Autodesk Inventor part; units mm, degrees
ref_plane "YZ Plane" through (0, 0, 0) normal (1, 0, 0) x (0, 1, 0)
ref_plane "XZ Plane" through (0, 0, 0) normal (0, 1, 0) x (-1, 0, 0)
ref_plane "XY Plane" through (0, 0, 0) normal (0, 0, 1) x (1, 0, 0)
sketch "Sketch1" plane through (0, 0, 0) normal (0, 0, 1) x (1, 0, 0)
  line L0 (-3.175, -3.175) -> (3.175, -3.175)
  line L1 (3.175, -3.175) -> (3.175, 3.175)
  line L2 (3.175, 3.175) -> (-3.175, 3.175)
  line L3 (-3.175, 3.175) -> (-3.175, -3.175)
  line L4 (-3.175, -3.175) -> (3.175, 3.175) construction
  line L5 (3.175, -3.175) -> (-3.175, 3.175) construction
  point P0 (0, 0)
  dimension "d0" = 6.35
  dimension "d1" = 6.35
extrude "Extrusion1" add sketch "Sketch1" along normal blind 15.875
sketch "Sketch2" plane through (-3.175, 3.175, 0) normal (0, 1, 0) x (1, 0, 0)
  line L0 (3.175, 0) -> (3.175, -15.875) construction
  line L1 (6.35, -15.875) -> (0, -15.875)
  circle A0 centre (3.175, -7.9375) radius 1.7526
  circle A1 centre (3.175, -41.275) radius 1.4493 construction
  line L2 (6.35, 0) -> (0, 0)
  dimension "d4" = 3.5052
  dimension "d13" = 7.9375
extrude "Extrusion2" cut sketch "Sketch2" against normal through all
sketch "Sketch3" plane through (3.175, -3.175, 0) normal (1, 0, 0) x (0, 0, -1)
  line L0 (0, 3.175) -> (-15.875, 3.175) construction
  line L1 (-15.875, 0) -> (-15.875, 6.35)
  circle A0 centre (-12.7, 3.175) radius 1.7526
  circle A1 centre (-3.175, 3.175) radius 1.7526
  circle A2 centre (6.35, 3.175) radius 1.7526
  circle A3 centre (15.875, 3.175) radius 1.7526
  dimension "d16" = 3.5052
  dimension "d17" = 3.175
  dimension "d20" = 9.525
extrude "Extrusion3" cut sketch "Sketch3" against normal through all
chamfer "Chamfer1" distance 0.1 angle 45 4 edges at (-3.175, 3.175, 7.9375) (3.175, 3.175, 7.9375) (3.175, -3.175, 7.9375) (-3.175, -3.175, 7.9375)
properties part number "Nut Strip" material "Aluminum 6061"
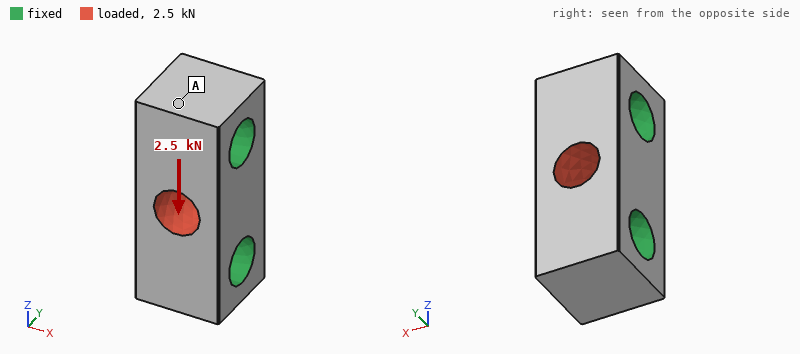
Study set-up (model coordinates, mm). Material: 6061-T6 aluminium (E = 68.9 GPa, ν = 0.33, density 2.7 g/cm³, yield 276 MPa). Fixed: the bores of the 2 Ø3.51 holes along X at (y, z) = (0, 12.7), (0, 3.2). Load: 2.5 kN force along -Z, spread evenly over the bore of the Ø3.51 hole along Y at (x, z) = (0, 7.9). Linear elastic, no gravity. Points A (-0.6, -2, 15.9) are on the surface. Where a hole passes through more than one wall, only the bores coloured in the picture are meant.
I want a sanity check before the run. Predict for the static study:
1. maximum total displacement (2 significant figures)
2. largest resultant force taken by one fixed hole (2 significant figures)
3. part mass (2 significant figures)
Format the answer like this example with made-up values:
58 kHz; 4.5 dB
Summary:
1.9 µm; 1.3 kN; 1.2 g
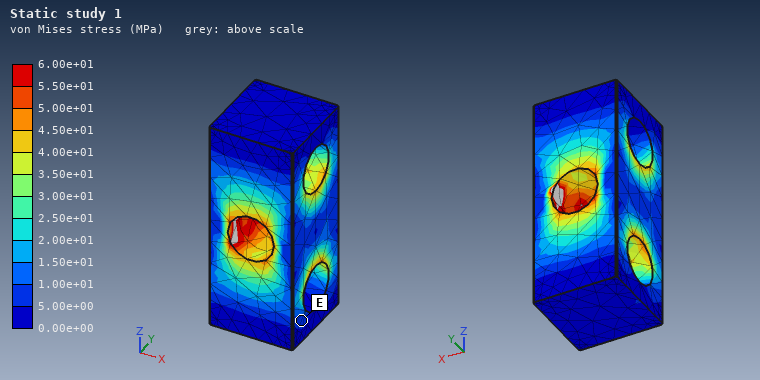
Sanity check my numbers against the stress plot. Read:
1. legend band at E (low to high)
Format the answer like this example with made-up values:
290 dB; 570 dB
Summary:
5.00e+00 to 1.00e+01 MPa
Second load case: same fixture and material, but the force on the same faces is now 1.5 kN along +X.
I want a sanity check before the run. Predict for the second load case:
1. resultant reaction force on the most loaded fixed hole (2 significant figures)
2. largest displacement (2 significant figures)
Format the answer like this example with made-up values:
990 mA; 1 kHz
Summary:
750 N; 3.5 µm
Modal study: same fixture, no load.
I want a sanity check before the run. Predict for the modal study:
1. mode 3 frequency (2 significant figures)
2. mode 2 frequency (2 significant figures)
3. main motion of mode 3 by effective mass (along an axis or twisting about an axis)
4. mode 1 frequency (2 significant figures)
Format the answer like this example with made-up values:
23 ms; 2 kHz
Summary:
220 kHz; 210 kHz; along X; 200 kHz
